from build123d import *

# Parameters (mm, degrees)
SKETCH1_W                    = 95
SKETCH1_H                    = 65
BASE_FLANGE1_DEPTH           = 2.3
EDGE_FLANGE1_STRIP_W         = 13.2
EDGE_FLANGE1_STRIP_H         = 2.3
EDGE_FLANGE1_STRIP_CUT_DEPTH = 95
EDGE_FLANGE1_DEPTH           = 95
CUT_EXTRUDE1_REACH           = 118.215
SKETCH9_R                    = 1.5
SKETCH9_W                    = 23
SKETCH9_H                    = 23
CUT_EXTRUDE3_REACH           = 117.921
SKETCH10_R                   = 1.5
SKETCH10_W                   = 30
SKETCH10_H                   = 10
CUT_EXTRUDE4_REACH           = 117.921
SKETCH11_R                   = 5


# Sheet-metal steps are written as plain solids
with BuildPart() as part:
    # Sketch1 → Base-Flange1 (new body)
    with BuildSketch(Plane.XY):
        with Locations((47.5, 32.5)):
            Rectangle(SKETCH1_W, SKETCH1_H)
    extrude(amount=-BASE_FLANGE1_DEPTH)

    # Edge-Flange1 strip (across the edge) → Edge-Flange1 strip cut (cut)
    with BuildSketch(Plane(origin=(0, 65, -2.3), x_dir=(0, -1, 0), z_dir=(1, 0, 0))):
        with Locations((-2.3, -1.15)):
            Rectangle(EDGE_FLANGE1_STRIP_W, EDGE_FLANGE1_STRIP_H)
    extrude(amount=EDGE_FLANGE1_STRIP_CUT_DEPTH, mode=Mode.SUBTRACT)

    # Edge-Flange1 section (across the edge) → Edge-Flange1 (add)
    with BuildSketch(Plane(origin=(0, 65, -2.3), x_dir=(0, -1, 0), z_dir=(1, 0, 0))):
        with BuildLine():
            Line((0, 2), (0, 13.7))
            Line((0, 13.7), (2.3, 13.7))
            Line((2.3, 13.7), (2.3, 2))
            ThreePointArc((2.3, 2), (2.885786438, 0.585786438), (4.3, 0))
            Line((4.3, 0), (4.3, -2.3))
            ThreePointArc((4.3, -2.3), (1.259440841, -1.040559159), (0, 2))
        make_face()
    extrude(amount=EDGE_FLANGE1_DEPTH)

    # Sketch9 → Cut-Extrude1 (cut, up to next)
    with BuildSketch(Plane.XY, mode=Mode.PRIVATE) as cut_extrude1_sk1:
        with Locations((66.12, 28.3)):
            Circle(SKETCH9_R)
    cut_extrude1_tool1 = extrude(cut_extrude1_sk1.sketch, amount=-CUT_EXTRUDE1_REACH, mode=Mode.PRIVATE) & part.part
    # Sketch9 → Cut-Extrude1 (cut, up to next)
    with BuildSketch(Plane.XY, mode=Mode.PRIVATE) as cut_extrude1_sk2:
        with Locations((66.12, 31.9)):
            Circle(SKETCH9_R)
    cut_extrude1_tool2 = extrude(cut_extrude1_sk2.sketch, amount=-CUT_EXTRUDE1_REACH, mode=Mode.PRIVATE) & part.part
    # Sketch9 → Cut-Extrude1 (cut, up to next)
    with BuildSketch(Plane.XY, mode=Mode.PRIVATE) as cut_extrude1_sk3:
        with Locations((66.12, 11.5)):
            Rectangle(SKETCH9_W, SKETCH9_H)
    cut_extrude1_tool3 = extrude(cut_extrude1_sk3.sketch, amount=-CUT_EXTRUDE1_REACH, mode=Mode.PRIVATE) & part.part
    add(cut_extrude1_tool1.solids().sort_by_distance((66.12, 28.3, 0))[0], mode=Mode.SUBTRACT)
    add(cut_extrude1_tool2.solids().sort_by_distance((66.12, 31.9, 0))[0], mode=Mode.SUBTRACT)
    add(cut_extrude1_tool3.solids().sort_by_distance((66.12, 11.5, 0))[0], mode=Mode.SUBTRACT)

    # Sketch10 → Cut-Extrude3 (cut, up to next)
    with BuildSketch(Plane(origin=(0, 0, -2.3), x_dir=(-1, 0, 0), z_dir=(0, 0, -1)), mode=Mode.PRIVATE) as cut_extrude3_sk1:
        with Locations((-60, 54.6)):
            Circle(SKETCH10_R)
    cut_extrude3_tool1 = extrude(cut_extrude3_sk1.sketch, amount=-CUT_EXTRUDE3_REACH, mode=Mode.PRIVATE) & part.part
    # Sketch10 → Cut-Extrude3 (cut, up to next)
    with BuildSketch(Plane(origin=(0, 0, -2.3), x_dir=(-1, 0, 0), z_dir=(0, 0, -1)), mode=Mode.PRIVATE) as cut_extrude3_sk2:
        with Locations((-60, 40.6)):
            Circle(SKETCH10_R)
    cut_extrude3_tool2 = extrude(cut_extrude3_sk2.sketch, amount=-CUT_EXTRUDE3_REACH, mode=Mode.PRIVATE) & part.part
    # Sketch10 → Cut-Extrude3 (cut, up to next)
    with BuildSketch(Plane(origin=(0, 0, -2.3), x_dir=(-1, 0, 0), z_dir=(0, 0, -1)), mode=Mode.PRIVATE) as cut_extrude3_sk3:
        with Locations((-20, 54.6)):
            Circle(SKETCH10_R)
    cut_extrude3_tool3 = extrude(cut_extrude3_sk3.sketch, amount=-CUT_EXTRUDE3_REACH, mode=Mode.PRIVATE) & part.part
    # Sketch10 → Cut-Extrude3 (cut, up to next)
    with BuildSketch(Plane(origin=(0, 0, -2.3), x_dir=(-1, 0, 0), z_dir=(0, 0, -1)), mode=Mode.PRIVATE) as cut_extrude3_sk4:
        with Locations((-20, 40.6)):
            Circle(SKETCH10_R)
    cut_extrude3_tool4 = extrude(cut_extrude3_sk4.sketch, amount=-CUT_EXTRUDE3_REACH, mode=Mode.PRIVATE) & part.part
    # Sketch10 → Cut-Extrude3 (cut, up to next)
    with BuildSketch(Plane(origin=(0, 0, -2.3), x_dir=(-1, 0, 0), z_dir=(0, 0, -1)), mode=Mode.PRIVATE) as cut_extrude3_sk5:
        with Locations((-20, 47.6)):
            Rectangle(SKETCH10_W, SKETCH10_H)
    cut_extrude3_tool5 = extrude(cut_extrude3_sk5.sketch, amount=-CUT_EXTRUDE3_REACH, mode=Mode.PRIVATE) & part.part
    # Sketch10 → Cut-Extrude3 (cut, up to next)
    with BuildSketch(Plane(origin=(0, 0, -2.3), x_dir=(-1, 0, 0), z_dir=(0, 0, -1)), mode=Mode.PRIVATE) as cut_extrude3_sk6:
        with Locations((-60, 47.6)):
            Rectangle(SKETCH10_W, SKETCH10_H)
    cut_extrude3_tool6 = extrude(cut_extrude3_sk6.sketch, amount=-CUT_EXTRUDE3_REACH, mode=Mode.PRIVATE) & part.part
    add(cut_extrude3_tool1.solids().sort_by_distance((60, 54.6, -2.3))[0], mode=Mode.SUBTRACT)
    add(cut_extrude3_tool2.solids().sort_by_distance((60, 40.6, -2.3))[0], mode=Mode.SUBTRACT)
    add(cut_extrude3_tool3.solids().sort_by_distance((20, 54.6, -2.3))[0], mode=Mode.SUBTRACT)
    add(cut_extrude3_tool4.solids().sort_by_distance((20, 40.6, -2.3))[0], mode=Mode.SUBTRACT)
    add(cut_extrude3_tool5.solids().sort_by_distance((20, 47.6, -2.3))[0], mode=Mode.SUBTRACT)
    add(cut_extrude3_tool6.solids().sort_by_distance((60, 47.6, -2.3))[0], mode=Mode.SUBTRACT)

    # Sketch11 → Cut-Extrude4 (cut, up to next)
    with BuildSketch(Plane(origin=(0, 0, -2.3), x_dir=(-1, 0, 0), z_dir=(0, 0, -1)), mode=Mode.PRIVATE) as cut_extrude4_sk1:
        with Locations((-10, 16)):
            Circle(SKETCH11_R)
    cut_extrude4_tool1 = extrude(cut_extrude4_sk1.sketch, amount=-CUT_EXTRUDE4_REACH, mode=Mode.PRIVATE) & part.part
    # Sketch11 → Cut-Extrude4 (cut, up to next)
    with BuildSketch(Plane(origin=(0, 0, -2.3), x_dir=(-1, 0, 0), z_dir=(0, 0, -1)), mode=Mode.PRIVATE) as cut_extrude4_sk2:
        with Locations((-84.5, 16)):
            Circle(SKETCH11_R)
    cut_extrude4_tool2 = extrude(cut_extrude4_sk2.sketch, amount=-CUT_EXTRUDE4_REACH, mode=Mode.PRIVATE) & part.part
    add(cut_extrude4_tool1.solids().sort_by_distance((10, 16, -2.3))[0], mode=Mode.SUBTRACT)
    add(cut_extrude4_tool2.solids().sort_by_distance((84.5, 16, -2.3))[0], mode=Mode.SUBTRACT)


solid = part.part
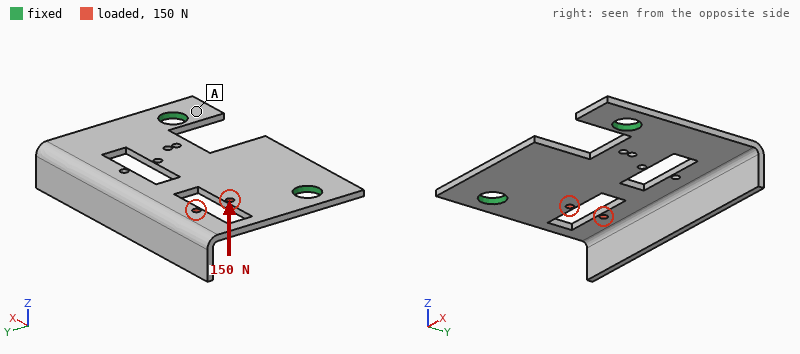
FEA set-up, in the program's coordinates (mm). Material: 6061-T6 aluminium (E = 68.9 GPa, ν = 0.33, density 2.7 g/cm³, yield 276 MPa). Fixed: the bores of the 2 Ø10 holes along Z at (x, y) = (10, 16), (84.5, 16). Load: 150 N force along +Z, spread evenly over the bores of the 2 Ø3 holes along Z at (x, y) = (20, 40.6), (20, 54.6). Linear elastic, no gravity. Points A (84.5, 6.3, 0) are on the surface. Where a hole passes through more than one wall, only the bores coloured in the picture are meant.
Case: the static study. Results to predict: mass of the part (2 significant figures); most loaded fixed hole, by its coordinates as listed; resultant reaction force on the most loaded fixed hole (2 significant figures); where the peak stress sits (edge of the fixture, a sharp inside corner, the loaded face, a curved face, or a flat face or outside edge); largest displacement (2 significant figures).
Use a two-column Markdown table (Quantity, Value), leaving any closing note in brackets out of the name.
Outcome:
| Quantity | Value |
|---|---|
| mass of the part | 37 g |
| most loaded fixed hole, by its coordinates as listed | (10, 16) |
| resultant reaction force on the most loaded fixed hole | 130 N |
| where the peak stress sits | a flat face or outside edge |
| largest displacement | 0.82 mm |
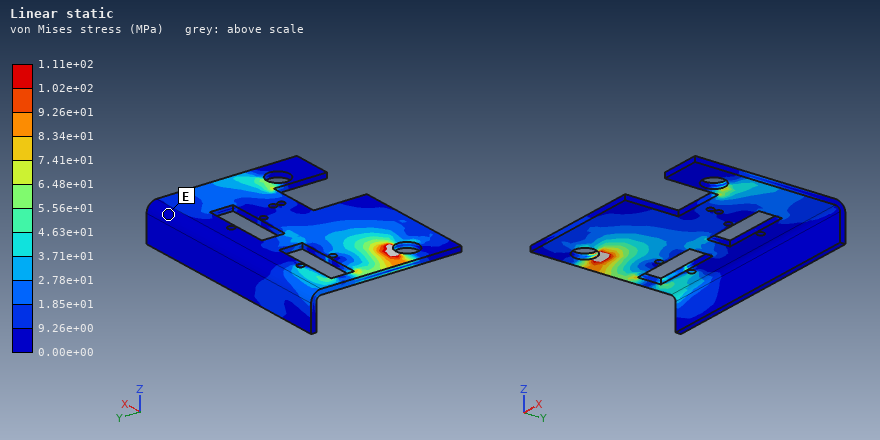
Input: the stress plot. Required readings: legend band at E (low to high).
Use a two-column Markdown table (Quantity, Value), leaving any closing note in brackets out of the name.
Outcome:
| Quantity | Value |
|---|---|
| legend band at E | 0.00e+00 to 9.26e+00 MPa |
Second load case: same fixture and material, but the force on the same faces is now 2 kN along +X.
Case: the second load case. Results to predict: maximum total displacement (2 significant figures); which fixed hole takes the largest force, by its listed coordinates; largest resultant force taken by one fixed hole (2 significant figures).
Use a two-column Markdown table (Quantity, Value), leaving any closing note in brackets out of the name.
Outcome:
| Quantity | Value |
|---|---|
| maximum total displacement | 59 µm |
| which fixed hole takes the largest force, by its listed coordinates | (10, 16) |
| largest resultant force taken by one fixed hole | 1.5 kN |
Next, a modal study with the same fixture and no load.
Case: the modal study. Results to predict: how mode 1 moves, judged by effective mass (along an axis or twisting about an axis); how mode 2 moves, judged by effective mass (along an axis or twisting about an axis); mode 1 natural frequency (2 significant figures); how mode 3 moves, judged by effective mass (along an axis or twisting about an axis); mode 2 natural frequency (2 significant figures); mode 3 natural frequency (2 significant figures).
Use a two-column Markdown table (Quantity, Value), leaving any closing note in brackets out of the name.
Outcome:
| Quantity | Value |
|---|---|
| how mode 1 moves, judged by effective mass | along Z |
| how mode 2 moves, judged by effective mass | twisting about Y |
| mode 1 natural frequency | 480 Hz |
| how mode 3 moves, judged by effective mass | along Z |
| mode 2 natural frequency | 970 Hz |
| mode 3 natural frequency | 1900 Hz |
